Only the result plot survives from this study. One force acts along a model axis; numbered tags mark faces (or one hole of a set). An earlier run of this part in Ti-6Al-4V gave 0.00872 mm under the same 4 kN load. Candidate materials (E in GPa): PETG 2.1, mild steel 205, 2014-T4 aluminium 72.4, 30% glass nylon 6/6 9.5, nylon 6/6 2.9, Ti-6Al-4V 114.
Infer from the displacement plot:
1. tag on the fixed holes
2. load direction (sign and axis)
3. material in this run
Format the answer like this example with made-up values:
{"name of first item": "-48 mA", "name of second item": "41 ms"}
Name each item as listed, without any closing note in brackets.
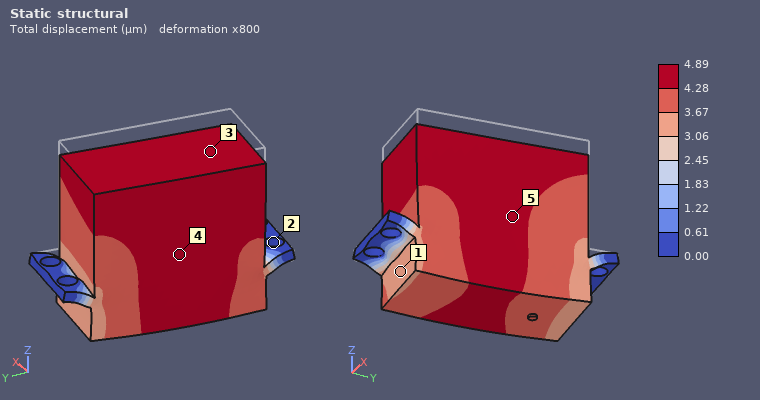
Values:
{"tag on the fixed holes": "2", "load direction": "-Z", "material in this run": "mild steel"}
